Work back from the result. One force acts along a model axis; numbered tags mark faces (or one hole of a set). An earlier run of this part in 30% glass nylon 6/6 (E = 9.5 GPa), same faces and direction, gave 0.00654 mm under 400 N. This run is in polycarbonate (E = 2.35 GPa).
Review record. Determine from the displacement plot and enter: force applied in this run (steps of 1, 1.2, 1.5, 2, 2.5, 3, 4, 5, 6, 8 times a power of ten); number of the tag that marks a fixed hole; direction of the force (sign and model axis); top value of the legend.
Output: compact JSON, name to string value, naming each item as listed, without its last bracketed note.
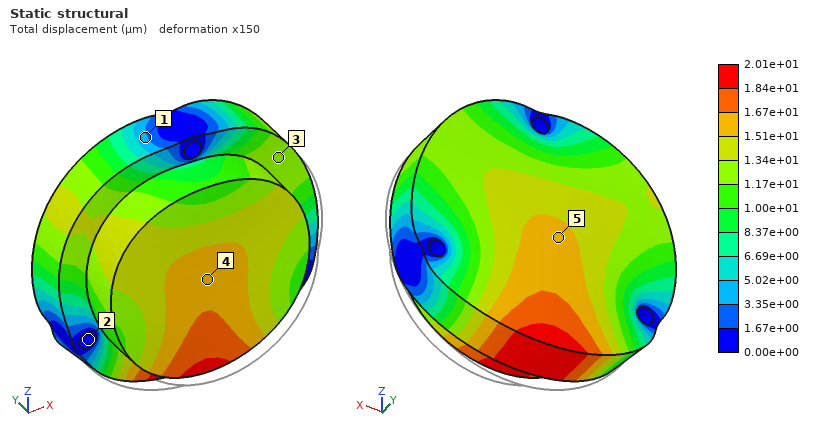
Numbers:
{"force applied in this run": "300 N", "number of the tag that marks a fixed hole": "2", "direction of the force": "+Y", "top value of the legend": "2.01e+01 µm"}
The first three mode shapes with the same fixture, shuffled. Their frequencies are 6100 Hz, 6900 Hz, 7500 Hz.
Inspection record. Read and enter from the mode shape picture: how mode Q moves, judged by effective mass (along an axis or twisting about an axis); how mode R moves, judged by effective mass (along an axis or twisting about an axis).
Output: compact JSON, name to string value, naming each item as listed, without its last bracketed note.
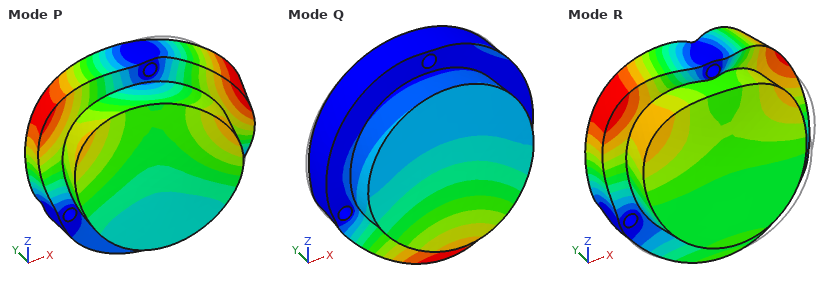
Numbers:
{"how mode Q moves, judged by effective mass": "along Y", "how mode R moves, judged by effective mass": "along Y"}
